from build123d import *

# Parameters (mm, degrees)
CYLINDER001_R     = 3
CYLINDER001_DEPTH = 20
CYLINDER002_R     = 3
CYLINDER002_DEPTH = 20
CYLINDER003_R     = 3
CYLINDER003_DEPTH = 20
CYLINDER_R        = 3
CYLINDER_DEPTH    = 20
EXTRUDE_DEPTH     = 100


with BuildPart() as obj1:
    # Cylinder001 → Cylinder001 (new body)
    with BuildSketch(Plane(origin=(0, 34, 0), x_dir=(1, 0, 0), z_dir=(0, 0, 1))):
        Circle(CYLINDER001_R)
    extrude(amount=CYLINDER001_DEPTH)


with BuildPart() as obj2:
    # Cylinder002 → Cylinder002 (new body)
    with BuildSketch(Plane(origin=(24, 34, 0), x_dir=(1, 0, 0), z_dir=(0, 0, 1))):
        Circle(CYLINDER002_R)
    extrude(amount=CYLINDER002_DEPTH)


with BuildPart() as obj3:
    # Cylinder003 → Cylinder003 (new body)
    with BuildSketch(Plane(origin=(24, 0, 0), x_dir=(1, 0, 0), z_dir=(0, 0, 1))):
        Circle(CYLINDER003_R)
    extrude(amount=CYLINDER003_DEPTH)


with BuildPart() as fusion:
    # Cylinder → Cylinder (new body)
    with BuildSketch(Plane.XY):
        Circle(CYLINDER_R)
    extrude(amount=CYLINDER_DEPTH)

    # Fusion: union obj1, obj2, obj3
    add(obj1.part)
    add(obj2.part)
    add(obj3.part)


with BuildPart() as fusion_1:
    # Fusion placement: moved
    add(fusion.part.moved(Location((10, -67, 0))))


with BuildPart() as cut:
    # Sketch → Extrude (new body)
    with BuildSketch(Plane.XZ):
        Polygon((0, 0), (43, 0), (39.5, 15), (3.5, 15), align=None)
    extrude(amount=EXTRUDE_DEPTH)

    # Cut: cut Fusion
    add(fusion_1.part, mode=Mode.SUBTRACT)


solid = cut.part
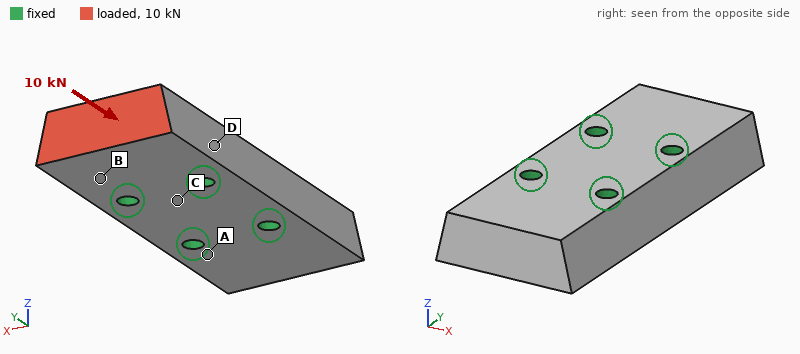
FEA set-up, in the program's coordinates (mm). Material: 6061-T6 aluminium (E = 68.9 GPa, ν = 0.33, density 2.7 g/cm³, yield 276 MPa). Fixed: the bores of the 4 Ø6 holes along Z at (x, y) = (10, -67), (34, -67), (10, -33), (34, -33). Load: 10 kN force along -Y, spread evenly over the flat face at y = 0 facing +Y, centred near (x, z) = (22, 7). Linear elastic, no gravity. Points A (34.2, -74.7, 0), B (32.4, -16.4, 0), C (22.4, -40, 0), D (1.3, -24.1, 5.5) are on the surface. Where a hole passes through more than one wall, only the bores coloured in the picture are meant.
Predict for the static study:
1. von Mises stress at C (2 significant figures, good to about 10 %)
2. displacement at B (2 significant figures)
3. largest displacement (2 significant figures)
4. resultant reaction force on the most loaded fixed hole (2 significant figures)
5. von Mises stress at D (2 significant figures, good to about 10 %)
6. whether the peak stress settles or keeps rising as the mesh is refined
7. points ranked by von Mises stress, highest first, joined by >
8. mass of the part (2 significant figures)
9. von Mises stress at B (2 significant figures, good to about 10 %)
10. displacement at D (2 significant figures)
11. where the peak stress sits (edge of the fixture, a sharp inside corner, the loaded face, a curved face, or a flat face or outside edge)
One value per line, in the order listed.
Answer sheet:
5.7 MPa
4.4 µm
8.8 µm
4.8 kN
13 MPa
keeps rising
B > D > C > A
160 g
18 MPa
3.2 µm
edge of the fixture
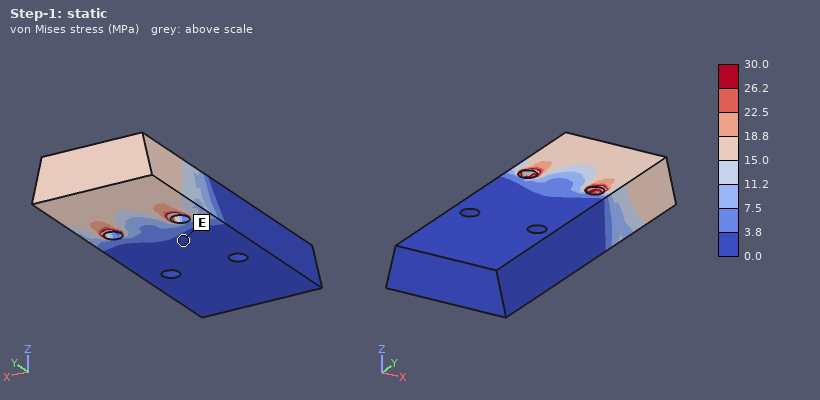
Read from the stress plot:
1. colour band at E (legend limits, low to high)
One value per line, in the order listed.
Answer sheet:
0.0 to 3.8 MPa
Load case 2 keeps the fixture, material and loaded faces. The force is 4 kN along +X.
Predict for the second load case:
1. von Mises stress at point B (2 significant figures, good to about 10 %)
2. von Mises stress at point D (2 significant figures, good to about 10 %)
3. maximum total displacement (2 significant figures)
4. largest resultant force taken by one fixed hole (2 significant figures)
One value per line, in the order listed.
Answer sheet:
16 MPa
21 MPa
24 µm
4.8 kN
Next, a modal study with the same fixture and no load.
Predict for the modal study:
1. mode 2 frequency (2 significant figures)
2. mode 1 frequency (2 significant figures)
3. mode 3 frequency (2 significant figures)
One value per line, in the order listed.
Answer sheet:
9900 Hz
9900 Hz
17 kHz
